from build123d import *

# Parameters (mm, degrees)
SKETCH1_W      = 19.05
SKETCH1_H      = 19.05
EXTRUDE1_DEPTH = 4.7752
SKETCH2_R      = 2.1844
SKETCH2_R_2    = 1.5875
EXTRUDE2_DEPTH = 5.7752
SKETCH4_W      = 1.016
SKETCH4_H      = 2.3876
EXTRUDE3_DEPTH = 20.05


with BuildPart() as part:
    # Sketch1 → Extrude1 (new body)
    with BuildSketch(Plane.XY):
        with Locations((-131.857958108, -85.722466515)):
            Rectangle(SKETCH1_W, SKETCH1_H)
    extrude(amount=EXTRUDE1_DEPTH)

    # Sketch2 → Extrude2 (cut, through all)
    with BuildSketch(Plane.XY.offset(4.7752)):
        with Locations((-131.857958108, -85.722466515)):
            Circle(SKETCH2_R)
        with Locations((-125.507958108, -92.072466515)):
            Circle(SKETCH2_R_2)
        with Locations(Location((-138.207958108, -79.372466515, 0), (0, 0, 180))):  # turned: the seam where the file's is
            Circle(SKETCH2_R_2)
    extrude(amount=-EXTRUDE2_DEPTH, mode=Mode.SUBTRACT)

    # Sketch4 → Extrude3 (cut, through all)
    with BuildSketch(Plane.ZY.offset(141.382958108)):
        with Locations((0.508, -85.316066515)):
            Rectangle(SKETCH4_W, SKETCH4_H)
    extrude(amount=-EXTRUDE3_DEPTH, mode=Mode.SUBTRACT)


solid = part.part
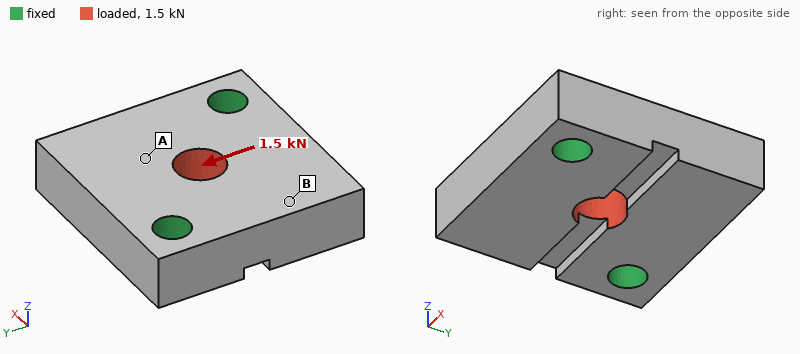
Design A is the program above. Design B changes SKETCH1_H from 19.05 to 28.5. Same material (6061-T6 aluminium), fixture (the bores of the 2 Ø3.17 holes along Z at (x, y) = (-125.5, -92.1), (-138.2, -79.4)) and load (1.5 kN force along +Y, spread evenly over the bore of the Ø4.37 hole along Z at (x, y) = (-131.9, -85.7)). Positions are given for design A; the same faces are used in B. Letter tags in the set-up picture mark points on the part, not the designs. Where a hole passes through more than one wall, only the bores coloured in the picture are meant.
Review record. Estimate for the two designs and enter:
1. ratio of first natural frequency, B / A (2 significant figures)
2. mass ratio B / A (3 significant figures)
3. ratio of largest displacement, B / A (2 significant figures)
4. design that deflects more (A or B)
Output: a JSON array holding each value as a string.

["0.74", "1.55", "0.89", "A"]
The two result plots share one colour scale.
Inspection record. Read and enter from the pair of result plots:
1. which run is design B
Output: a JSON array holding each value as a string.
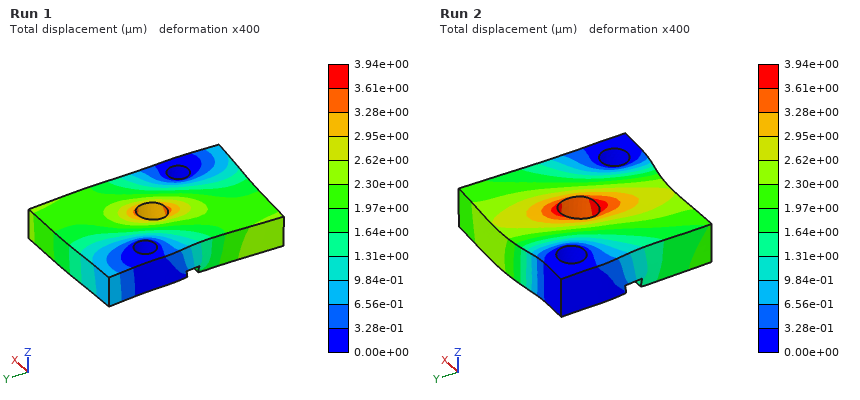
["Run 1"]
